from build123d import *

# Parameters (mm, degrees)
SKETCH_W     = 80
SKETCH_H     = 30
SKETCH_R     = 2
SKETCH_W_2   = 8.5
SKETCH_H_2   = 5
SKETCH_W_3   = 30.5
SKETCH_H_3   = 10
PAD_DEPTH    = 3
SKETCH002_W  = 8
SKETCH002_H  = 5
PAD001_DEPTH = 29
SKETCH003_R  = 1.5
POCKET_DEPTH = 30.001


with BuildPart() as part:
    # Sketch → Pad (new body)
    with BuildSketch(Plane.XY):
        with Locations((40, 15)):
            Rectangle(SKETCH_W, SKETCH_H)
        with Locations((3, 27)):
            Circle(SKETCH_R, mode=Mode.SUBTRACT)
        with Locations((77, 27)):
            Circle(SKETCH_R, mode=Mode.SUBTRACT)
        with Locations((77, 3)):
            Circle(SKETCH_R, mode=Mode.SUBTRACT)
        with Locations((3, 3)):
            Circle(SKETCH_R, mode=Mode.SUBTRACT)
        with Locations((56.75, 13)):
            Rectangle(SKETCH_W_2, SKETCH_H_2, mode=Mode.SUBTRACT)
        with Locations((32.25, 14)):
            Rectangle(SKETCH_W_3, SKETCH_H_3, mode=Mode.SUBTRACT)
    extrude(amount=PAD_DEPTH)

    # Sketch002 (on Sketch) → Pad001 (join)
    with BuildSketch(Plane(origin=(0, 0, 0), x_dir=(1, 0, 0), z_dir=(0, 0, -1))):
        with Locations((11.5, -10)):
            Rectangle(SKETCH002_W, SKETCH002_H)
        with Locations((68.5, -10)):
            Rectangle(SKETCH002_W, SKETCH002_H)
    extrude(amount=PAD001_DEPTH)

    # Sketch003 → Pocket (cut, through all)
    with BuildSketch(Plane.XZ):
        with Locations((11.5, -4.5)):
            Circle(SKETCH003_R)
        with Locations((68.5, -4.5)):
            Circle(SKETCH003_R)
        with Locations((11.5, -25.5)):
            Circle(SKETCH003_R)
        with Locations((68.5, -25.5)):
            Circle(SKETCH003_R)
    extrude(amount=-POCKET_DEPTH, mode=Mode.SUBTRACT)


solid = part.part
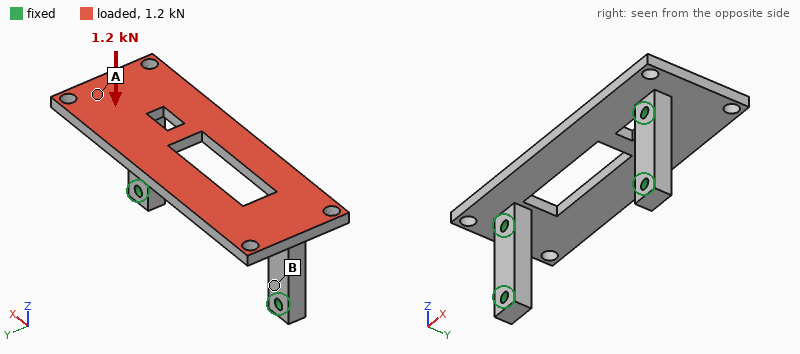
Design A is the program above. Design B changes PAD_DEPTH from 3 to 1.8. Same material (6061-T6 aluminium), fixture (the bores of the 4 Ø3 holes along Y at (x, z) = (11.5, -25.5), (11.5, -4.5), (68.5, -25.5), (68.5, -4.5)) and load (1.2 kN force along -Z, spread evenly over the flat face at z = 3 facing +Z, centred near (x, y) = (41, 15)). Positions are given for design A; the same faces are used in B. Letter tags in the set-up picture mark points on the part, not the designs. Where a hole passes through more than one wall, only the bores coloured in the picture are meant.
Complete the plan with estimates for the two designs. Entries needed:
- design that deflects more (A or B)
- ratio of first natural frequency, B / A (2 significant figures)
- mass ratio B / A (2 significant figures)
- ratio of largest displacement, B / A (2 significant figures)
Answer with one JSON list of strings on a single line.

["B", "0.70", "0.71", "3.6"]
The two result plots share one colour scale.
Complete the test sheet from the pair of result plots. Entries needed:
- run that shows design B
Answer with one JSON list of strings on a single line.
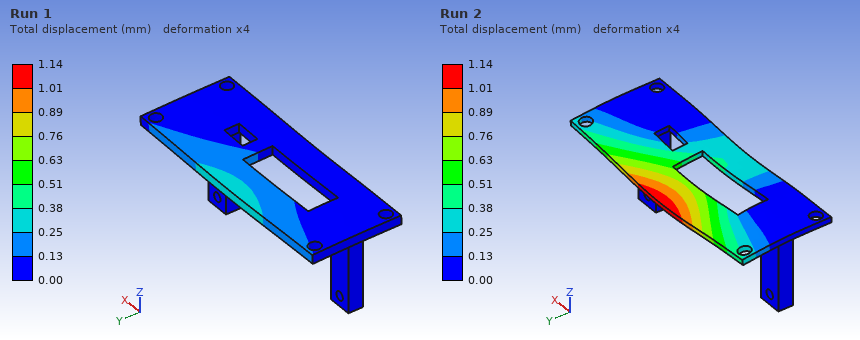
["Run 2"]
